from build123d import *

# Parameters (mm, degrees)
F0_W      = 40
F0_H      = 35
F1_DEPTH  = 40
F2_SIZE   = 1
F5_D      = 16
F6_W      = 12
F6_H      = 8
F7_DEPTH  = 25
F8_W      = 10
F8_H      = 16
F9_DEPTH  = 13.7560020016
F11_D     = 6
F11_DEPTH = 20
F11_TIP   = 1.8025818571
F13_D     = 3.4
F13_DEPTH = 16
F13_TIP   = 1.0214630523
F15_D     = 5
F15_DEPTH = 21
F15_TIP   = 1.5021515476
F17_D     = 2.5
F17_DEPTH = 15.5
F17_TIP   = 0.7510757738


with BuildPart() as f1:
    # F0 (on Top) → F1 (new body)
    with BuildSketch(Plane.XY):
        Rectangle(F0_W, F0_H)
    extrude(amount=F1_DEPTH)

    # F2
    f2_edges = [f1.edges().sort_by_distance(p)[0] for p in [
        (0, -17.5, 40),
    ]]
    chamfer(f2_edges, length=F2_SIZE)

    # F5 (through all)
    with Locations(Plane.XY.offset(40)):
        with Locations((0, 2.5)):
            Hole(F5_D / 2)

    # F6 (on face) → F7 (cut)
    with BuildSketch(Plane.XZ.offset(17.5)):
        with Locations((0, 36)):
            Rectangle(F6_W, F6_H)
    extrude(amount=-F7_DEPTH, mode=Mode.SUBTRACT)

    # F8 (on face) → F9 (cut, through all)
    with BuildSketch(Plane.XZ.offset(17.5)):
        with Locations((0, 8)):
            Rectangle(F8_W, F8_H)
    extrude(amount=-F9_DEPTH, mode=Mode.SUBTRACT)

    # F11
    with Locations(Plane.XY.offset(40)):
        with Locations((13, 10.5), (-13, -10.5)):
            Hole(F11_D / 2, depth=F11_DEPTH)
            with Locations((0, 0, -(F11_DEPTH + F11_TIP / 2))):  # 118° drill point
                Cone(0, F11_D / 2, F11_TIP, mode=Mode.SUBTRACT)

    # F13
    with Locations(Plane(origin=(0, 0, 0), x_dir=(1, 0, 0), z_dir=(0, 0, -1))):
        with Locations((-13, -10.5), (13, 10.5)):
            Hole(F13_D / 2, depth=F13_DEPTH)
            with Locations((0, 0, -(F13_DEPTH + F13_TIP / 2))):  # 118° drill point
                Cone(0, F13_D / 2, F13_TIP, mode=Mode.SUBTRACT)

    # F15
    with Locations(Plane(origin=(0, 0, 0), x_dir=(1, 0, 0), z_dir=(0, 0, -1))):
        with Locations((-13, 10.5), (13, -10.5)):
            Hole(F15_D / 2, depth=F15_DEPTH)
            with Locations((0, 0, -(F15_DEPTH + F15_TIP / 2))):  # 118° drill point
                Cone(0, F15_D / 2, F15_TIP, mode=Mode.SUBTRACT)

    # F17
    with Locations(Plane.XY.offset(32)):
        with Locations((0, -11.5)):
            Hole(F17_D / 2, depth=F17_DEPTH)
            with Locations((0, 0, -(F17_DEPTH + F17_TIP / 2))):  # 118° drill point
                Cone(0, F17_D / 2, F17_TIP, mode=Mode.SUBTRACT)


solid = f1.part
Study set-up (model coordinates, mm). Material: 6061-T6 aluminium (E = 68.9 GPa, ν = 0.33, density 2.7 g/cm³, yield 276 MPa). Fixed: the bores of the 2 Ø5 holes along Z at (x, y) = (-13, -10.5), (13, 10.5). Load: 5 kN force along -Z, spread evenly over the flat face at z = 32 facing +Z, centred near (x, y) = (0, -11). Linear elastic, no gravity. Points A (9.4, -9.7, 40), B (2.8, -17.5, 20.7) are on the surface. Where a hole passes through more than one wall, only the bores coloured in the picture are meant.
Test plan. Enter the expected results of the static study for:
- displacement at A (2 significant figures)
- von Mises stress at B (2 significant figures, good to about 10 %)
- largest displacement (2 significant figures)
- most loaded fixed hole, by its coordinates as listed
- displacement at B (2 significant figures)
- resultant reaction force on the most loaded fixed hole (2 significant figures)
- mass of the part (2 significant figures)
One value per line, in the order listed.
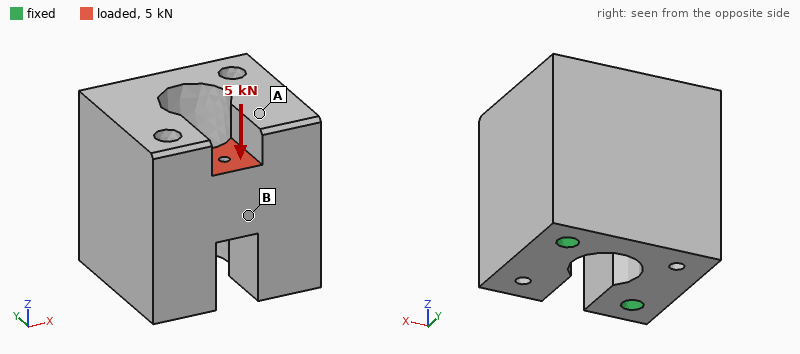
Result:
14 µm
12 MPa
18 µm
(-13, -10.5)
13 µm
3.3 kN
110 g
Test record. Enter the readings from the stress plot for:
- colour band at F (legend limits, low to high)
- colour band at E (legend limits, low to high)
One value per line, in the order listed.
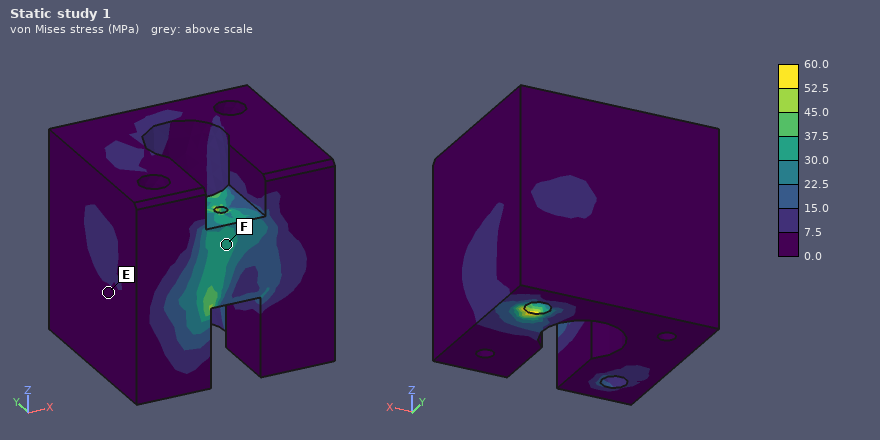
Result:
30.0 to 37.5 MPa
0.0 to 7.5 MPa
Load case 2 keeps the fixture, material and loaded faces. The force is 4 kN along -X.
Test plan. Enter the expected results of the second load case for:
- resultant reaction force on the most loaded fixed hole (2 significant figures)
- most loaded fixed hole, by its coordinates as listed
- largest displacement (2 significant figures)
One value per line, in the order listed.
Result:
3.4 kN
(-13, -10.5)
17 µm
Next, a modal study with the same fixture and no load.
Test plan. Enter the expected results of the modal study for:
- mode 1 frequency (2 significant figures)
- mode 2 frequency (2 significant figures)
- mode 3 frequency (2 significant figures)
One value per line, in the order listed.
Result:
9900 Hz
16 kHz
19 kHz
